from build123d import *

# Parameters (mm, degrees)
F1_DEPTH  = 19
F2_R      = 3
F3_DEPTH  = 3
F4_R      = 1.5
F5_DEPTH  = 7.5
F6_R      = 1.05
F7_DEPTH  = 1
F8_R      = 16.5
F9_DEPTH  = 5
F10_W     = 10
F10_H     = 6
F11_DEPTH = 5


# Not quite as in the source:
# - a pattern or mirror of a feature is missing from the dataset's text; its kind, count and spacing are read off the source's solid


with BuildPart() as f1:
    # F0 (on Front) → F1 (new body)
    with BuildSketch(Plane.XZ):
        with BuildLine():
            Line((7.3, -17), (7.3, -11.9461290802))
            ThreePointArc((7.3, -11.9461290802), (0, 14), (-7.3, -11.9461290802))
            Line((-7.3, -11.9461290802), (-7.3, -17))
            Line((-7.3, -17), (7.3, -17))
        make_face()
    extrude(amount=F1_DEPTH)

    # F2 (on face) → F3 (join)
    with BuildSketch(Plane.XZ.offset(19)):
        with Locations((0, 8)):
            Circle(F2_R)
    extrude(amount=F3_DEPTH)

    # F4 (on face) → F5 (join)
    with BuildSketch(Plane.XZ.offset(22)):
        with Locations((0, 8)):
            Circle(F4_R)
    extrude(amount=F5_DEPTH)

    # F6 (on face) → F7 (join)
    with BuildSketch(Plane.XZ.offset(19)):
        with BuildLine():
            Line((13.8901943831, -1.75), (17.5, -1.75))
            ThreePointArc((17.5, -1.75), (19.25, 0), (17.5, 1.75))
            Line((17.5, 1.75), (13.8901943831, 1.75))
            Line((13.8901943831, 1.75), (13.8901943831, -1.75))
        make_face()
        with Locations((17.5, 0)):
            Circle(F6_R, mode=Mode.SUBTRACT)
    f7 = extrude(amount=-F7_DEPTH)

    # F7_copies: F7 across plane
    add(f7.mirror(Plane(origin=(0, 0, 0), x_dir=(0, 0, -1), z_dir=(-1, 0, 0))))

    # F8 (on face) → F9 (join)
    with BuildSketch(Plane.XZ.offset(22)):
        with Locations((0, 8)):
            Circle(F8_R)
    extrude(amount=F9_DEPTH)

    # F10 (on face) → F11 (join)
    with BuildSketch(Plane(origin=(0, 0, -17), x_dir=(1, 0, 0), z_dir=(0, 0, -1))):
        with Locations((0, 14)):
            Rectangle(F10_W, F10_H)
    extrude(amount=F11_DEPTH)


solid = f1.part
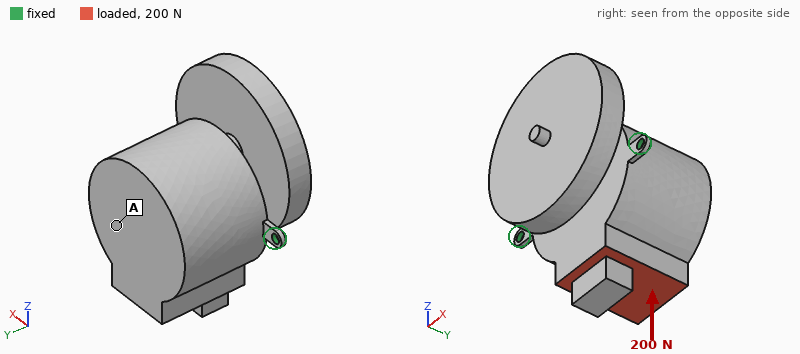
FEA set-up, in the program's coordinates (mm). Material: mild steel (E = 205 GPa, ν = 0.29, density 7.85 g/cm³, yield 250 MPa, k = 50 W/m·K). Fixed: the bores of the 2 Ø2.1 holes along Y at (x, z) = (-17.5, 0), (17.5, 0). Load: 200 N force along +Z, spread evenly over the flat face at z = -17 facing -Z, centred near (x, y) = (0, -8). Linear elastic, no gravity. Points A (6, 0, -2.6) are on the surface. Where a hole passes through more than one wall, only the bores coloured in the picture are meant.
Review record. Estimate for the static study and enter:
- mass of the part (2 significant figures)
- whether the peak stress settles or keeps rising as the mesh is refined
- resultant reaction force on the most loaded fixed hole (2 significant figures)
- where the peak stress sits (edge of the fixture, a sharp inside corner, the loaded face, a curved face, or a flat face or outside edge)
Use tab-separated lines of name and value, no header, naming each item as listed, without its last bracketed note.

mass of the part	140 g
whether the peak stress settles or keeps rising as the mesh is refined	keeps rising
resultant reaction force on the most loaded fixed hole	100 N
where the peak stress sits	edge of the fixture
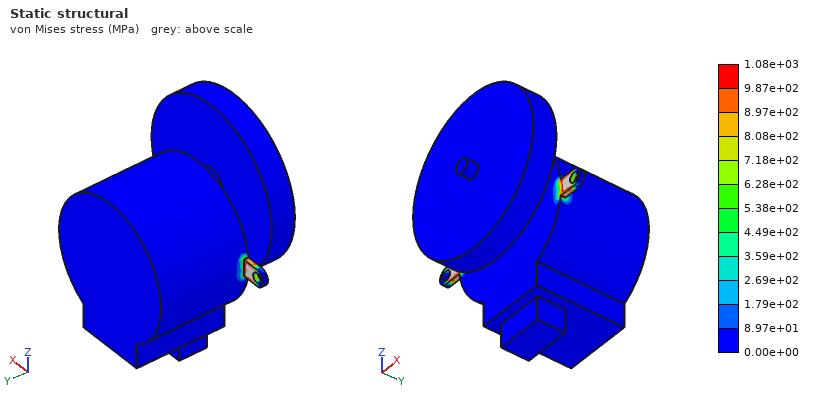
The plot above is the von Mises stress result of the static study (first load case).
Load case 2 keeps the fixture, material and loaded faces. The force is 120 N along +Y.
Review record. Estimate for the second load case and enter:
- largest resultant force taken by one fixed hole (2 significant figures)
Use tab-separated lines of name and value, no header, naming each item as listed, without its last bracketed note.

largest resultant force taken by one fixed hole	69 N
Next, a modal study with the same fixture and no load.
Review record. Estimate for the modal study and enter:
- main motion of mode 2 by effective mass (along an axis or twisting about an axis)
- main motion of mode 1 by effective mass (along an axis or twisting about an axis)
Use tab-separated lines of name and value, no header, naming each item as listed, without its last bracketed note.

main motion of mode 2 by effective mass	along Y
main motion of mode 1 by effective mass	along Z
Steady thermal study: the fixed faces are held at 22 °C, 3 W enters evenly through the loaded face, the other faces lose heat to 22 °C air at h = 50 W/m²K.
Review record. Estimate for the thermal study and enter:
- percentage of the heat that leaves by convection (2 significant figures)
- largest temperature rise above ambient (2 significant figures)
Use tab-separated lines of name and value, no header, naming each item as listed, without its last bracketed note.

percentage of the heat that leaves by convection	72 %
largest temperature rise above ambient	12 K
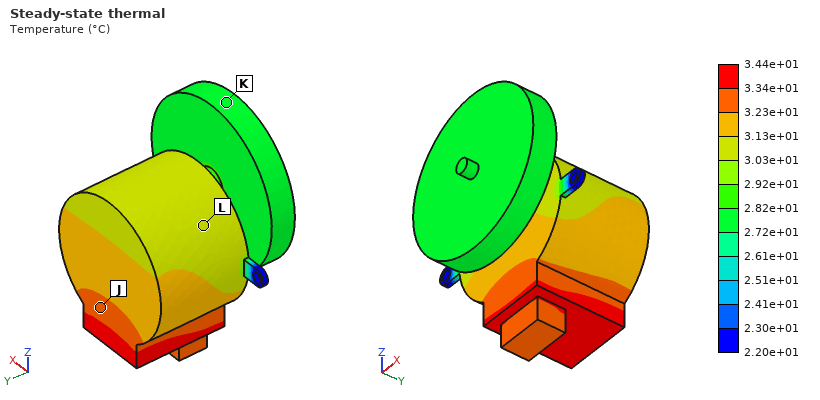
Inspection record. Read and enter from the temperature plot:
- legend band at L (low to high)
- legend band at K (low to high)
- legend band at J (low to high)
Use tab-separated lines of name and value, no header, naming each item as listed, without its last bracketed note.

legend band at L	3.03e+01 to 3.13e+01 °C
legend band at K	2.72e+01 to 2.82e+01 °C
legend band at J	3.23e+01 to 3.34e+01 °C
